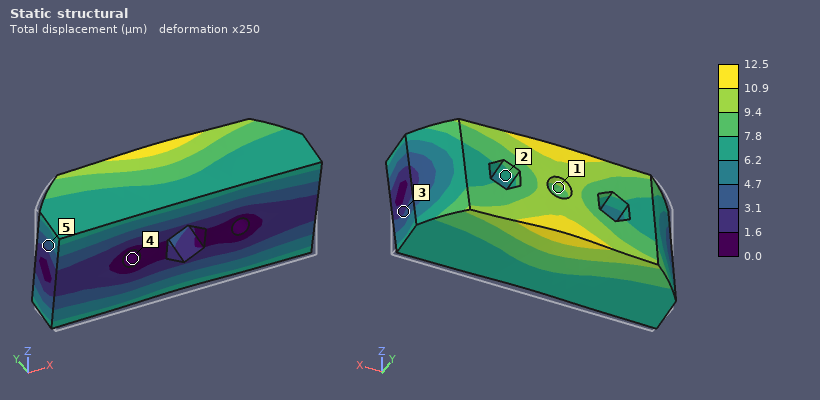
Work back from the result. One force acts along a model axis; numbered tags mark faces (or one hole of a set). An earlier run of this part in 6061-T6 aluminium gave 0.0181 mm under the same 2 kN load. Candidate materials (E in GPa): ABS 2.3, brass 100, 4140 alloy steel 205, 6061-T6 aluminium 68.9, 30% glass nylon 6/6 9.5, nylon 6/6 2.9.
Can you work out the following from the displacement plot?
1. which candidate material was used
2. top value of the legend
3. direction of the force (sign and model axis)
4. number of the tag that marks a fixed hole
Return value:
brass
12.5 µm
+Z
4
